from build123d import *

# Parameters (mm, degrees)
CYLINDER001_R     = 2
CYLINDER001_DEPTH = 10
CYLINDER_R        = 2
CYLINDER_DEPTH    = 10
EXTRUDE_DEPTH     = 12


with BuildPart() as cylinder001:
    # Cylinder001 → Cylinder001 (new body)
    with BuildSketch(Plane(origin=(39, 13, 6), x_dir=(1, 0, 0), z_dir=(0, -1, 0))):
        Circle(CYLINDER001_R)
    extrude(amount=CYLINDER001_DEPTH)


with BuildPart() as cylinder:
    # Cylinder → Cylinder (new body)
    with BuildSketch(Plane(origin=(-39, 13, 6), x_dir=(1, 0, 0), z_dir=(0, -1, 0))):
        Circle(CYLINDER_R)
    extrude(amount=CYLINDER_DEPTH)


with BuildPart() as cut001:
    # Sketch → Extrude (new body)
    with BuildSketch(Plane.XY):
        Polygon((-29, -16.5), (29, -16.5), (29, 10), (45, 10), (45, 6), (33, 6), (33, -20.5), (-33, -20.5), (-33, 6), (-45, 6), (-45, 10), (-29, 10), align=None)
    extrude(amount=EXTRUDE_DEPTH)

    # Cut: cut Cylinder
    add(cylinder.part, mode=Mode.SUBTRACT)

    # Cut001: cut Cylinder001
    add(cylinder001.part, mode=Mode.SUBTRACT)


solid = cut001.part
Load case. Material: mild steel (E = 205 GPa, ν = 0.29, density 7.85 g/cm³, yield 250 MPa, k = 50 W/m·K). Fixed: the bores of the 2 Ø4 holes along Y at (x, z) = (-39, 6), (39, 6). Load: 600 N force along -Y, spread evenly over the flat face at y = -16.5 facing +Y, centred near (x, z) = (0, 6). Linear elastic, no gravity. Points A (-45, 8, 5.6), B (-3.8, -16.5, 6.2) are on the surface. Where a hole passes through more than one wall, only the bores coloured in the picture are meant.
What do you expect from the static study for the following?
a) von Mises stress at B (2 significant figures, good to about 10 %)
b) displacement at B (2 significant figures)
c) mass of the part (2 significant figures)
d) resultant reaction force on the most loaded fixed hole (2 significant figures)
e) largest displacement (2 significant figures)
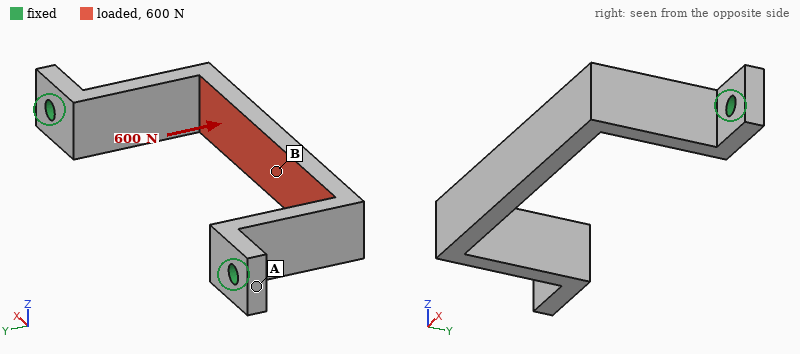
59 MPa
48 µm
53 g
340 N
50 µm
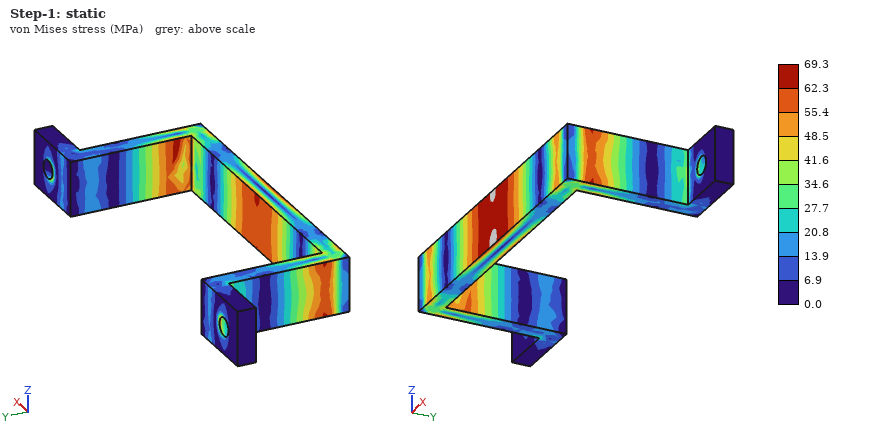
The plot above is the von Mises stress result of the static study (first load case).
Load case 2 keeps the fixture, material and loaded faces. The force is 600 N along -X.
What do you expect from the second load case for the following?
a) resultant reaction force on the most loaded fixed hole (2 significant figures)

320 N
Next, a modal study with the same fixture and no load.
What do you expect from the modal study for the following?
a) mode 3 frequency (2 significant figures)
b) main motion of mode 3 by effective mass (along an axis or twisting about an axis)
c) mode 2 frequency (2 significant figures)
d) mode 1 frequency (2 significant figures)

4000 Hz
twisting about Y
2400 Hz
2400 Hz
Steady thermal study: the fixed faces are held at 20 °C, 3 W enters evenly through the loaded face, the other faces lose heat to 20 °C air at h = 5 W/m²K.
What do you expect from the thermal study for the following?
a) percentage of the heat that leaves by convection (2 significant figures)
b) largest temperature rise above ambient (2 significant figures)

8.4 %
27 K
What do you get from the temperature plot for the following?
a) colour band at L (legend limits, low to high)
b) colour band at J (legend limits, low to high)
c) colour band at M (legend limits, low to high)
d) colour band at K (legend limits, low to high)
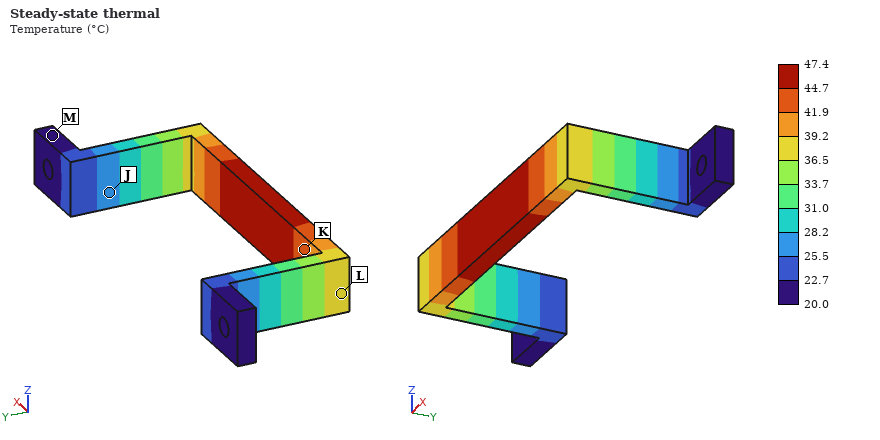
36.5 to 39.2 °C
25.5 to 28.2 °C
20.0 to 22.7 °C
41.9 to 44.7 °C
